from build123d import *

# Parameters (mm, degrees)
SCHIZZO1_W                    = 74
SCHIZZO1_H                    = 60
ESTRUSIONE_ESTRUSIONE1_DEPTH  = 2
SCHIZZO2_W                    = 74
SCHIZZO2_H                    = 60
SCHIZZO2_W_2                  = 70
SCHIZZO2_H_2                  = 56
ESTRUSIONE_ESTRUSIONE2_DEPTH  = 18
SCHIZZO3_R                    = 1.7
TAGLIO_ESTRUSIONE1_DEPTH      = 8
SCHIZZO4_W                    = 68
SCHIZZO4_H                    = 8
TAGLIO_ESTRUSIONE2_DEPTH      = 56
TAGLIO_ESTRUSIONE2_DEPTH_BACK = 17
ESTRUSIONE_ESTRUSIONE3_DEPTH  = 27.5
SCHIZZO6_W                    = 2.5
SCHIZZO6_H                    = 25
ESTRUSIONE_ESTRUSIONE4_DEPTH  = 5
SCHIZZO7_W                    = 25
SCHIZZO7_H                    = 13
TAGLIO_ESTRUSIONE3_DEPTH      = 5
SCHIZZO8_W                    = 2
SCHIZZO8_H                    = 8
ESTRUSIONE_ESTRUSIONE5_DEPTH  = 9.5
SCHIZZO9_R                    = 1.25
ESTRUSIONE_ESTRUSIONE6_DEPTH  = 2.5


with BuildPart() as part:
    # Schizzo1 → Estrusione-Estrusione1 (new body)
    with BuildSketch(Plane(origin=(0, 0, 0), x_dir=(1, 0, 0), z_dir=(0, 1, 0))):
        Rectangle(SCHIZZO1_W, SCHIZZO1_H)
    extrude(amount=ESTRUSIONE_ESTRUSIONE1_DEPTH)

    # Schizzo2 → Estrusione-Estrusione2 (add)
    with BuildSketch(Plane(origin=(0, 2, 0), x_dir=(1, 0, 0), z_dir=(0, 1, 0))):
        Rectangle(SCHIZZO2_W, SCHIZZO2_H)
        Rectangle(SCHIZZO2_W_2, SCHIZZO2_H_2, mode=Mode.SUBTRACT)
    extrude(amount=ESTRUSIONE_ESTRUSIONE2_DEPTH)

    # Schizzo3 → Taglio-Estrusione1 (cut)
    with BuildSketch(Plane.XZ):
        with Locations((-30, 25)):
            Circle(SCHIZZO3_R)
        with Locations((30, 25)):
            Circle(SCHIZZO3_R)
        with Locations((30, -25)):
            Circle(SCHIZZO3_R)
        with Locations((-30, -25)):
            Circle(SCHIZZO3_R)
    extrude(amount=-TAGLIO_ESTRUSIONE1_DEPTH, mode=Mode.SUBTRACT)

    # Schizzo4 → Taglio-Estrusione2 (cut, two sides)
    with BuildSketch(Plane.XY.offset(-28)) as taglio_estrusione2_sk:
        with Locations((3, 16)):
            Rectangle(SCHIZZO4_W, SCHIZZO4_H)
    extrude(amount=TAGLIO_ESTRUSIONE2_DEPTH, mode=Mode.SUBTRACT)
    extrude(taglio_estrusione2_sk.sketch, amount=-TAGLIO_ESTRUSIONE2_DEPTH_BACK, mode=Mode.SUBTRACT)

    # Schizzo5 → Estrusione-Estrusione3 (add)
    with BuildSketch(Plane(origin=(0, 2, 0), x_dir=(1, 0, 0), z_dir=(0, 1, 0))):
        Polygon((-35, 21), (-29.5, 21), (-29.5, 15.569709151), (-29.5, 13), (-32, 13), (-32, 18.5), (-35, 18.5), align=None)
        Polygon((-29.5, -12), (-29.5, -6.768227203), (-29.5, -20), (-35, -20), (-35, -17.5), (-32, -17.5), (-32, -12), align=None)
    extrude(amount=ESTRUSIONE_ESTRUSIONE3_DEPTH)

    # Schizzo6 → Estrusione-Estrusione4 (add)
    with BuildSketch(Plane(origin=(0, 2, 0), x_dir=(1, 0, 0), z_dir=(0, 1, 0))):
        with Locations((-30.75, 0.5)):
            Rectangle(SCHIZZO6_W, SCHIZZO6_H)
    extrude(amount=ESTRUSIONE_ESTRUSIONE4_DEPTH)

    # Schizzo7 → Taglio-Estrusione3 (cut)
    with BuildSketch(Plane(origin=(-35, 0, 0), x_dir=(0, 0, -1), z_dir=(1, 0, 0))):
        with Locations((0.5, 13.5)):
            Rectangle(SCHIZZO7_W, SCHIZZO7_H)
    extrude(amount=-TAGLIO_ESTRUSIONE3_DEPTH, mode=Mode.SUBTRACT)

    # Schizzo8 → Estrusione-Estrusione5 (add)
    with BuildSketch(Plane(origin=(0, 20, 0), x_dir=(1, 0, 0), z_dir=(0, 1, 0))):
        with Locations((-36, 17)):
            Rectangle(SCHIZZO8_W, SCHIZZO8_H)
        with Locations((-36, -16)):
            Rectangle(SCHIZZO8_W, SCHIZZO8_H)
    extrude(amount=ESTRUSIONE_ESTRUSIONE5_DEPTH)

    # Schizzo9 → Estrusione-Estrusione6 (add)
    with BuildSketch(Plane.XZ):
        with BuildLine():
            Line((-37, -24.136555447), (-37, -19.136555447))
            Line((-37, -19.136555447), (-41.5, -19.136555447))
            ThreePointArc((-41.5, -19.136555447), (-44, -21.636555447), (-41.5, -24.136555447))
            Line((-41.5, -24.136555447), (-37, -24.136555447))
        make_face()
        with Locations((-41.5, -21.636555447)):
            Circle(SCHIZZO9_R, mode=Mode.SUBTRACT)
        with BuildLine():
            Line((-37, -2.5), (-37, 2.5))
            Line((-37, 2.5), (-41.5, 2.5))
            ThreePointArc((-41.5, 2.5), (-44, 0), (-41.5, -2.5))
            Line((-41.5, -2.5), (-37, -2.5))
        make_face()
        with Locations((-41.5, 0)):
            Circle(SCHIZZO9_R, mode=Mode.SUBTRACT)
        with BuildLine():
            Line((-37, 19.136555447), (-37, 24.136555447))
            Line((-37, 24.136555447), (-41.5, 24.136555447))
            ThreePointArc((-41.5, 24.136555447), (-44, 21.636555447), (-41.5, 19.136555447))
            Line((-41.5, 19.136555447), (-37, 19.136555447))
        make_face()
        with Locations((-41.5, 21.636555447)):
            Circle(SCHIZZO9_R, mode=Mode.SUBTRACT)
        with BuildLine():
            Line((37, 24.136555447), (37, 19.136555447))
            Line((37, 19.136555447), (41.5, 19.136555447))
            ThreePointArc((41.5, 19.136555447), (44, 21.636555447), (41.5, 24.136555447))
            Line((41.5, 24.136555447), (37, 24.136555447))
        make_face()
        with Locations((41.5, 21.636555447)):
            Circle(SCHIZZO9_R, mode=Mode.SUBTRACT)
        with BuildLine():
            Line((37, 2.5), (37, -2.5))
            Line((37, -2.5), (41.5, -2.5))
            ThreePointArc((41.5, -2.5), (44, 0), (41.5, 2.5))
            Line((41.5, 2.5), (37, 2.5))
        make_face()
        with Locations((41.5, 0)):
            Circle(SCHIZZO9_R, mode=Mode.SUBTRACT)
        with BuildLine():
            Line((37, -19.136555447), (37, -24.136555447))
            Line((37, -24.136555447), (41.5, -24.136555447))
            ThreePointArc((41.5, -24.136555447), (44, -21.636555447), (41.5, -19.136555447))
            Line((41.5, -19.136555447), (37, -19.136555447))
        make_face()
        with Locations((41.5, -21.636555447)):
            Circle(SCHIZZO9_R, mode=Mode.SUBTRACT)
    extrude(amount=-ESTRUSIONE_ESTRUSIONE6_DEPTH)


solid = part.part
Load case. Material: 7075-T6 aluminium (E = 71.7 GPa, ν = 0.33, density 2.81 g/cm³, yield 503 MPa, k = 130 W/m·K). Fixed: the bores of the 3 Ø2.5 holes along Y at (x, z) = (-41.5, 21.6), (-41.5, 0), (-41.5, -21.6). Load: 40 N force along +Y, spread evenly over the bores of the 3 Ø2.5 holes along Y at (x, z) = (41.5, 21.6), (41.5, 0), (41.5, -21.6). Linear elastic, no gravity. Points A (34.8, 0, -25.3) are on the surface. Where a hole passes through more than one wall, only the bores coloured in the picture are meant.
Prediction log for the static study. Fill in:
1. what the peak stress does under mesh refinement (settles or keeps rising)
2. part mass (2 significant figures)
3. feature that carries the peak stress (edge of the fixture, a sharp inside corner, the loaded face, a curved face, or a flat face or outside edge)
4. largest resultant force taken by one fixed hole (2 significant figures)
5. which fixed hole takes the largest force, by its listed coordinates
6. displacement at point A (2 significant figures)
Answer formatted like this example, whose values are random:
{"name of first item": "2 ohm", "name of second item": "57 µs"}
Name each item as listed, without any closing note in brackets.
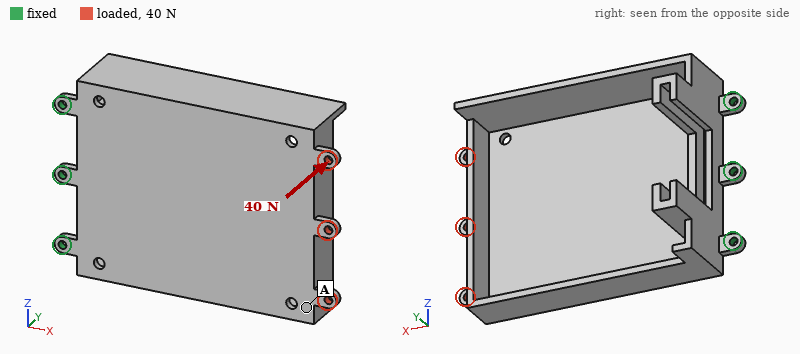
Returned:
{"what the peak stress does under mesh refinement": "keeps rising", "part mass": "51 g", "feature that carries the peak stress": "edge of the fixture", "largest resultant force taken by one fixed hole": "98 N", "which fixed hole takes the largest force, by its listed coordinates": "(-41.5, 0)", "displacement at point A": "0.95 mm"}
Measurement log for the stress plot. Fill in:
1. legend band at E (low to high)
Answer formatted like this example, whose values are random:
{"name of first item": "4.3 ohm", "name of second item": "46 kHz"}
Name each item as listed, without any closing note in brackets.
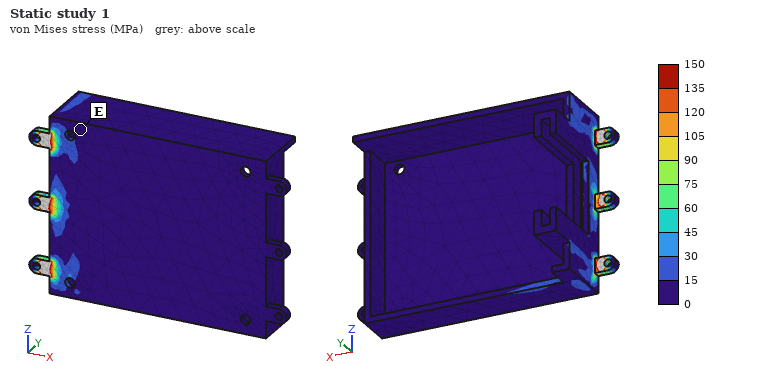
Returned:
{"legend band at E": "0 to 15 MPa"}
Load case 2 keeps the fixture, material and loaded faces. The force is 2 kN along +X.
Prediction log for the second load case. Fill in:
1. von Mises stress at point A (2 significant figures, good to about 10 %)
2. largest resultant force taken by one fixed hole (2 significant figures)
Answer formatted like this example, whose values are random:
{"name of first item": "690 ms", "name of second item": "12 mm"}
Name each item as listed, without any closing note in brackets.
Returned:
{"von Mises stress at point A": "26 MPa", "largest resultant force taken by one fixed hole": "680 N"}
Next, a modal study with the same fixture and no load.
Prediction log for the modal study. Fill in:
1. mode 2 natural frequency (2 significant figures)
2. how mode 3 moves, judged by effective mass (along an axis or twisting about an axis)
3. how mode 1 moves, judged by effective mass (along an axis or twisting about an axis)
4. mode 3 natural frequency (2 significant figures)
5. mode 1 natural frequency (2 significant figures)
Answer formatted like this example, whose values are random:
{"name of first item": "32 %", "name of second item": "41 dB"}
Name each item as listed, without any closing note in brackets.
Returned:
{"mode 2 natural frequency": "720 Hz", "how mode 3 moves, judged by effective mass": "along Z", "how mode 1 moves, judged by effective mass": "along Y", "mode 3 natural frequency": "3000 Hz", "mode 1 natural frequency": "260 Hz"}
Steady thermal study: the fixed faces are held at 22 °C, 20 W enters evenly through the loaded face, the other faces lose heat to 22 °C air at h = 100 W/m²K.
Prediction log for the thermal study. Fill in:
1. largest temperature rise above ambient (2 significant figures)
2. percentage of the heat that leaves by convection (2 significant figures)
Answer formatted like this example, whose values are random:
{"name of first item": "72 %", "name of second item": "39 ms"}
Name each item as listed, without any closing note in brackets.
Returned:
{"largest temperature rise above ambient": "56 K", "percentage of the heat that leaves by convection": "90 %"}
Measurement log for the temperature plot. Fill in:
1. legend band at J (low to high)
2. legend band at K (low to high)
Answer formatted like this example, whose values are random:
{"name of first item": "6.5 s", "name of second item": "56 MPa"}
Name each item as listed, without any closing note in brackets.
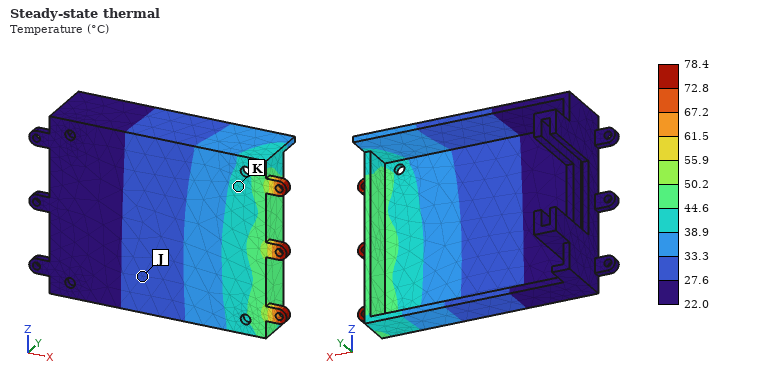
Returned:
{"legend band at J": "27.6 to 33.3 °C", "legend band at K": "38.9 to 44.6 °C"}
